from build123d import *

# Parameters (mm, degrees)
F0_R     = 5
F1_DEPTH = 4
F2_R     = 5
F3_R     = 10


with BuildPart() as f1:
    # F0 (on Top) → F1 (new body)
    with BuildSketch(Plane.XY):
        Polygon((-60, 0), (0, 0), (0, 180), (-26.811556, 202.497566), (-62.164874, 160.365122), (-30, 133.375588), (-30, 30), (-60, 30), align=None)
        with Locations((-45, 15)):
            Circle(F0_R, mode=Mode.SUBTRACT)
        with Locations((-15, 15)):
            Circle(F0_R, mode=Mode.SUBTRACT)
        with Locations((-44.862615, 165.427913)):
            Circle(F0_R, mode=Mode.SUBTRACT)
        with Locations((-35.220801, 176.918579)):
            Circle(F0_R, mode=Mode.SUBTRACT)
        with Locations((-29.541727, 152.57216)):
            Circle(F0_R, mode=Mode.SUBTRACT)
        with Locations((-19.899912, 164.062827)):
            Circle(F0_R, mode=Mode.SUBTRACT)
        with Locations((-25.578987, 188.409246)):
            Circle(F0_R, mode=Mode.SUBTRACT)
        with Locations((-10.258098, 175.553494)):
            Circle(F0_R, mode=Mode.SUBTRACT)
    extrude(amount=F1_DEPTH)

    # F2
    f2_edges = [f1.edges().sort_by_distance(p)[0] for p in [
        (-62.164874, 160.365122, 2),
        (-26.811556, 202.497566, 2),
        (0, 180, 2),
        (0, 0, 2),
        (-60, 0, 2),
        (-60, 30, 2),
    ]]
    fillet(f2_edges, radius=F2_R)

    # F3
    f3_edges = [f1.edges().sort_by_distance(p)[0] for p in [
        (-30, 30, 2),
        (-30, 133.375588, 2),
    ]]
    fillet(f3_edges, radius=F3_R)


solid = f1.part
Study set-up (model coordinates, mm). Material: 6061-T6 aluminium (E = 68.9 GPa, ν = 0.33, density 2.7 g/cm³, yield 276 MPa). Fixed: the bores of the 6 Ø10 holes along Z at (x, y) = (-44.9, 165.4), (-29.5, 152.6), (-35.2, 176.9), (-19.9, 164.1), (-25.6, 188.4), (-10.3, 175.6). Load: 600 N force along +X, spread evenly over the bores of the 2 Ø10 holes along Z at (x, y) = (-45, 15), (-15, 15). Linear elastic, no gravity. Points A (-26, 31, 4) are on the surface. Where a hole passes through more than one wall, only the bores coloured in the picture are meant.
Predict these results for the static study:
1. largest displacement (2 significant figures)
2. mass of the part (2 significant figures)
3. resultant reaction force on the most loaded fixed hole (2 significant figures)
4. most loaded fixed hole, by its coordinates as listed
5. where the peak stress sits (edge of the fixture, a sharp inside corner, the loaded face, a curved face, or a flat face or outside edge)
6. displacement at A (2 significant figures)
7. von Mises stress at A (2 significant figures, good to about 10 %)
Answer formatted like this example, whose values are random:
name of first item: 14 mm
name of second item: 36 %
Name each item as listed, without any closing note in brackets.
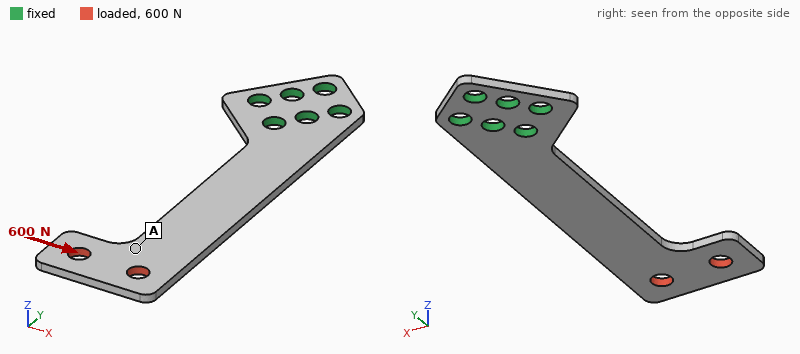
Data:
largest displacement: 0.99 mm
mass of the part: 77 g
resultant reaction force on the most loaded fixed hole: 2.6 kN
most loaded fixed hole, by its coordinates as listed: (-29.5, 152.6)
where the peak stress sits: a curved face
displacement at A: 0.66 mm
von Mises stress at A: 12 MPa
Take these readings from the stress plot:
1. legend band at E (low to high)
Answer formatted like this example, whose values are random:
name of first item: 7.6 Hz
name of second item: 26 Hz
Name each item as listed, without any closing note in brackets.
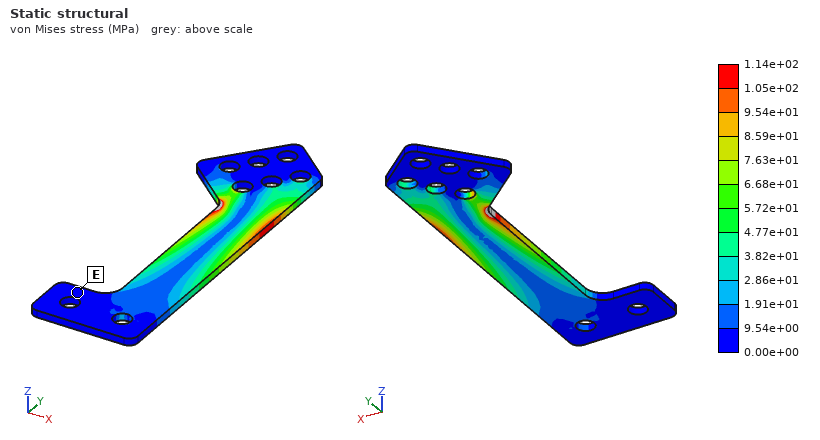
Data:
legend band at E: 0.00e+00 to 9.54e+00 MPa
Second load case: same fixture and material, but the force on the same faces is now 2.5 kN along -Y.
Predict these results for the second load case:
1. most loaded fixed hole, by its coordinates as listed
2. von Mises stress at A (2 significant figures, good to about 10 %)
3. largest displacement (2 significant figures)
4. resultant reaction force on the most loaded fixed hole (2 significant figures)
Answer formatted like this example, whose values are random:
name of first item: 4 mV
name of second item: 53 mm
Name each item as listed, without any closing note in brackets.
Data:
most loaded fixed hole, by its coordinates as listed: (-29.5, 152.6)
von Mises stress at A: 40 MPa
largest displacement: 0.71 mm
resultant reaction force on the most loaded fixed hole: 2.0 kN
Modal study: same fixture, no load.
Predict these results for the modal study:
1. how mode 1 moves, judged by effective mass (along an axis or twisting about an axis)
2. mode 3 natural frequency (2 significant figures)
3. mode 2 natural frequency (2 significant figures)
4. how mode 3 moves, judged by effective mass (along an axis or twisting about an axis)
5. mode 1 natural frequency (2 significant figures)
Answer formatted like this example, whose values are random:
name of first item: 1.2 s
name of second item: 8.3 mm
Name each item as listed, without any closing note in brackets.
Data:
how mode 1 moves, judged by effective mass: along Z
mode 3 natural frequency: 870 Hz
mode 2 natural frequency: 600 Hz
how mode 3 moves, judged by effective mass: along X
mode 1 natural frequency: 120 Hz
